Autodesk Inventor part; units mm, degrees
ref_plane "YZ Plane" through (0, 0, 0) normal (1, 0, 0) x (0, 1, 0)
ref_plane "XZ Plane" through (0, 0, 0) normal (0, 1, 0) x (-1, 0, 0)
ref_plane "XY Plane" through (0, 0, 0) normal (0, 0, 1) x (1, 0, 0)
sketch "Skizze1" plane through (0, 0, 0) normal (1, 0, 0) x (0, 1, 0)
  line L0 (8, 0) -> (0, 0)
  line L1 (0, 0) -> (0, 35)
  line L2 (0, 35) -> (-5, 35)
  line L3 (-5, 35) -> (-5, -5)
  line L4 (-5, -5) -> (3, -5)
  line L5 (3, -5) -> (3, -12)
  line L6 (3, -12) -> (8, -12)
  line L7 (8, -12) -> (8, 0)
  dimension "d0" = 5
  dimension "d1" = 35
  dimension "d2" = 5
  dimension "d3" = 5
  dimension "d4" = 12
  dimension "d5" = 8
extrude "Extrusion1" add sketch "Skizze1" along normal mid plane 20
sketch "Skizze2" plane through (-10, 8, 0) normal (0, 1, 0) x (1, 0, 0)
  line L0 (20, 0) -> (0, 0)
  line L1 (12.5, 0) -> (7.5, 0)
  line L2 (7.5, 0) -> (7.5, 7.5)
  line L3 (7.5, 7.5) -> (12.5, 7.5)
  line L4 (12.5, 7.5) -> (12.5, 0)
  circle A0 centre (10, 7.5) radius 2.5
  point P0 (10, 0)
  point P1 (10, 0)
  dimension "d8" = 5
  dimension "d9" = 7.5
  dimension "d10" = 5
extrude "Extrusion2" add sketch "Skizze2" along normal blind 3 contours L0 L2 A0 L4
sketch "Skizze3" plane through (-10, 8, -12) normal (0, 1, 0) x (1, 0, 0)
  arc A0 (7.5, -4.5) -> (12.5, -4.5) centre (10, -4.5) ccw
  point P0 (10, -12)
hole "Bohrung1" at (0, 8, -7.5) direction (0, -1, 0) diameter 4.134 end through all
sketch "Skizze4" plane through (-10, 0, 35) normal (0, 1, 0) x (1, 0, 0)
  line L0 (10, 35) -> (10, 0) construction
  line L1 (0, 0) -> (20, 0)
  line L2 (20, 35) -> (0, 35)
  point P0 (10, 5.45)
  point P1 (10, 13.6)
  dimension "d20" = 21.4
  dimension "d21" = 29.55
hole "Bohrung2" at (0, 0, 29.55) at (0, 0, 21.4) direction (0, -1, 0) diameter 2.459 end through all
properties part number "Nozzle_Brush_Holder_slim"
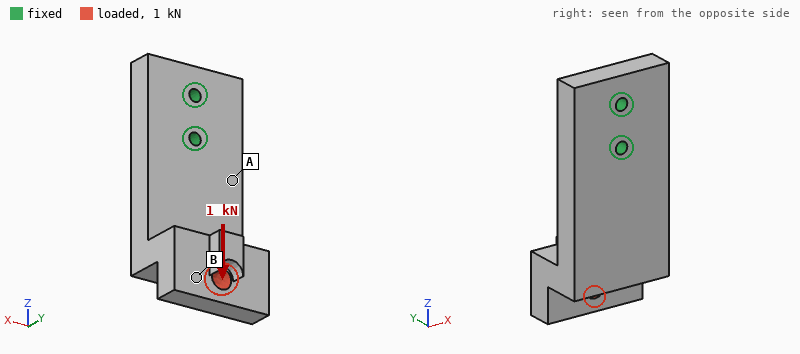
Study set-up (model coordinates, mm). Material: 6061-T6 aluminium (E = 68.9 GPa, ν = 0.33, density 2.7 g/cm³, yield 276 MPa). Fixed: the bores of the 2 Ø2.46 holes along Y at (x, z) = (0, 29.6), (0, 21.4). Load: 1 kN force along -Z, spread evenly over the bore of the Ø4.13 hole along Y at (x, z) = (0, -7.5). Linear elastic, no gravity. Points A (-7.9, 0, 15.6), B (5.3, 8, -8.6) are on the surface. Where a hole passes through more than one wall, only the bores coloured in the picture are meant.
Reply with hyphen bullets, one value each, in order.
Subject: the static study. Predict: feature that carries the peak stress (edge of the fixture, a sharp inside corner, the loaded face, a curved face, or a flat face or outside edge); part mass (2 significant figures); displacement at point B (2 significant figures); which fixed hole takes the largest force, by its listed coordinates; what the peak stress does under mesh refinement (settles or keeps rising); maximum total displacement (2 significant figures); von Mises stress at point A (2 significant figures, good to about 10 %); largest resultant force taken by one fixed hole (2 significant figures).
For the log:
- edge of the fixture
- 15 g
- 0.31 mm
- (0, 21.4)
- keeps rising
- 0.35 mm
- 97 MPa
- 840 N
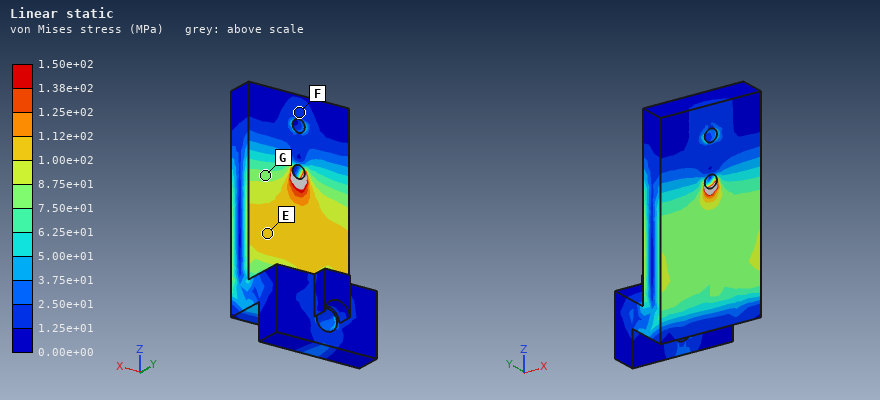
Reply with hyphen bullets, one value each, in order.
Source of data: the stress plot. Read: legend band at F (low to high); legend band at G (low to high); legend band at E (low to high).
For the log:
- 1.25e+01 to 2.50e+01 MPa
- 7.50e+01 to 8.75e+01 MPa
- 1.00e+02 to 1.12e+02 MPa
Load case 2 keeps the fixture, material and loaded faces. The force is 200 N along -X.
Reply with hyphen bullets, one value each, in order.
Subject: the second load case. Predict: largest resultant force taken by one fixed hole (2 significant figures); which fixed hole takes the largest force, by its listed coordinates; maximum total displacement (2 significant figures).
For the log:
- 730 N
- (0, 21.4)
- 48 µm
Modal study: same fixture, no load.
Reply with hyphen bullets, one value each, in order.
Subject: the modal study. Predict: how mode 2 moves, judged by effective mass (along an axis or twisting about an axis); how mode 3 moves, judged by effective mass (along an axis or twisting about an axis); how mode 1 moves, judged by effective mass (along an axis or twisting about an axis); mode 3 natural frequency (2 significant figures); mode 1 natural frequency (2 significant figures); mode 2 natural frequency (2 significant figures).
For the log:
- along X
- along X
- along Y
- 9100 Hz
- 2800 Hz
- 5300 Hz
